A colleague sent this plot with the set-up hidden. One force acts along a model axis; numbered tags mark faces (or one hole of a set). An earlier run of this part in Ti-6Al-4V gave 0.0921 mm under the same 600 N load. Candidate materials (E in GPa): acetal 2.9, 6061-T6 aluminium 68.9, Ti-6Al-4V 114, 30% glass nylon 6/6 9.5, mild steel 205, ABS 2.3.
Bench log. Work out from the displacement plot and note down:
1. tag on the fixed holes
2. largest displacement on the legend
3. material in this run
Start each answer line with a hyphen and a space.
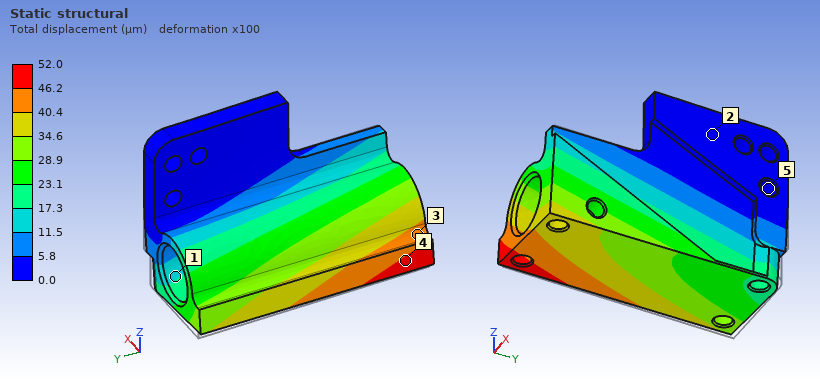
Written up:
- 5
- 52.0 µm
- mild steel
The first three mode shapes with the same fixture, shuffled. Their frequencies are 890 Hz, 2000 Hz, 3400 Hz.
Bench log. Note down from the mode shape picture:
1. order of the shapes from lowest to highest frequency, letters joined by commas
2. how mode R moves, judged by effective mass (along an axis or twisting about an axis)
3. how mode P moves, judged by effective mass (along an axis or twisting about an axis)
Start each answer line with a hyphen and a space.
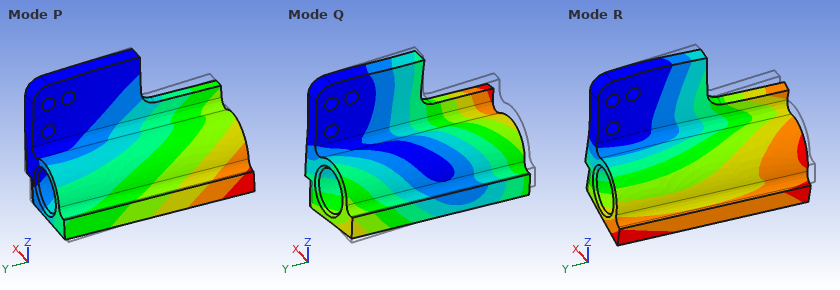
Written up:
- P, R, Q
- along Z
- along X
